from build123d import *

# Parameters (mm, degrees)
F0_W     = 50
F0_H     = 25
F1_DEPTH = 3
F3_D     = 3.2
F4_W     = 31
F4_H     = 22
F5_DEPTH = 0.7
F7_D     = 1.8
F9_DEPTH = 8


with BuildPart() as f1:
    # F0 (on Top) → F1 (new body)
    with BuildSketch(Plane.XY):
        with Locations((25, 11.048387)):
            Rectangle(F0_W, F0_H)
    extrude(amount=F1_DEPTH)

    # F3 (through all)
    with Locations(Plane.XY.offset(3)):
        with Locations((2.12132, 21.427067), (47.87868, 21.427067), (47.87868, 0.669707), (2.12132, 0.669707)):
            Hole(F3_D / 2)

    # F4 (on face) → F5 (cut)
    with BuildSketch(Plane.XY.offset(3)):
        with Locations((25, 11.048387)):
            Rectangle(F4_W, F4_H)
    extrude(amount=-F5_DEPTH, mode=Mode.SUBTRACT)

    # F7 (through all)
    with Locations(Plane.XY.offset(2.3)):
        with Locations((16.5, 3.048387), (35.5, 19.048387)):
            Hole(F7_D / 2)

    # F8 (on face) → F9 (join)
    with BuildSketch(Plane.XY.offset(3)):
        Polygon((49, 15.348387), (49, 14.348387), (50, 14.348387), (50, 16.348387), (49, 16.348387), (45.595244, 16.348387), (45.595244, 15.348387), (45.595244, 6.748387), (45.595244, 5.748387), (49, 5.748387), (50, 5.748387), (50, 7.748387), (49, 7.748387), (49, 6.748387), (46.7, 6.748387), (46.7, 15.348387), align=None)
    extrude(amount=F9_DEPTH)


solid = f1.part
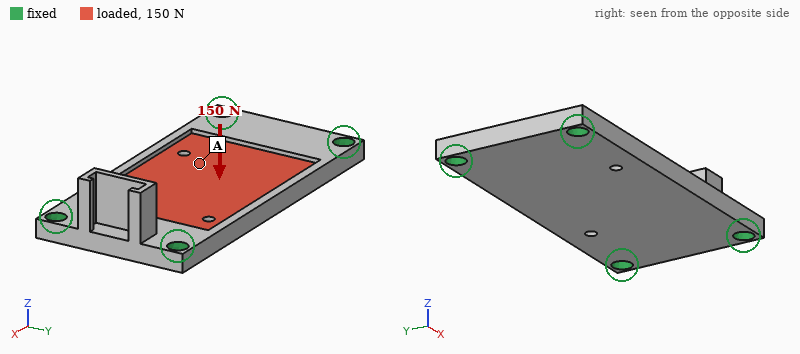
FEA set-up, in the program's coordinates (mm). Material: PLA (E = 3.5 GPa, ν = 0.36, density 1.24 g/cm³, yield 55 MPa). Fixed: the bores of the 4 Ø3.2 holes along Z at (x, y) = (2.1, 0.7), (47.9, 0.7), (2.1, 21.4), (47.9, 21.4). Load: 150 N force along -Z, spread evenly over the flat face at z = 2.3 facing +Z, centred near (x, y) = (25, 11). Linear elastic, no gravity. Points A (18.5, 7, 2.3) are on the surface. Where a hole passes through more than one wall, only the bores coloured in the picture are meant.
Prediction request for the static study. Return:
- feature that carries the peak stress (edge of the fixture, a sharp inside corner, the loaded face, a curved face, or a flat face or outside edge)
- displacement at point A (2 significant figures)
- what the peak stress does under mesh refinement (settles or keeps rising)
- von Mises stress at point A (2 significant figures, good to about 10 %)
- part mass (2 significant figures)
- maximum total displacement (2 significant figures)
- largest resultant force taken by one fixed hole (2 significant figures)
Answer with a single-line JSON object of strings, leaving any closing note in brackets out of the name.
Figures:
{"feature that carries the peak stress": "edge of the fixture", "displacement at point A": "0.33 mm", "what the peak stress does under mesh refinement": "keeps rising", "von Mises stress at point A": "8.0 MPa", "part mass": "4.1 g", "maximum total displacement": "0.39 mm", "largest resultant force taken by one fixed hole": "46 N"}
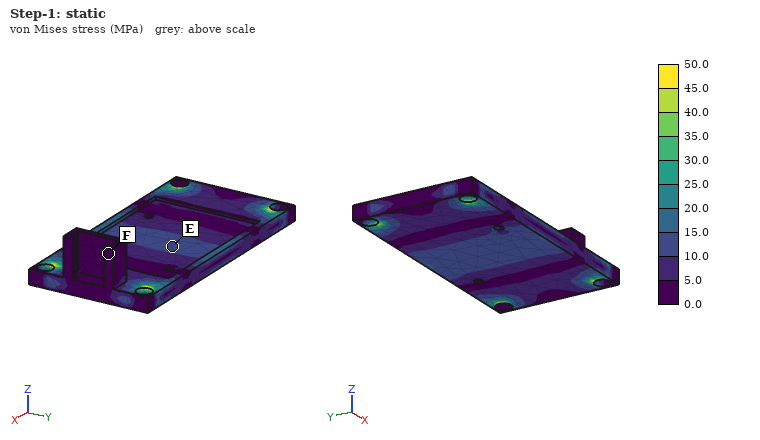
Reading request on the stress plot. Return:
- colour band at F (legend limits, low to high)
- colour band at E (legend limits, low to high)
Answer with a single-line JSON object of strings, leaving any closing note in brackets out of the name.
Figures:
{"colour band at F": "0.0 to 5.0 MPa", "colour band at E": "10.0 to 15.0 MPa"}
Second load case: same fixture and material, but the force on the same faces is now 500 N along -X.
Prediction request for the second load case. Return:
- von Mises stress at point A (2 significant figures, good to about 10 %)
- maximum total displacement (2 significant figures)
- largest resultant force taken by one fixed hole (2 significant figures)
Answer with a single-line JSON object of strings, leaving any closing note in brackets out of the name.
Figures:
{"von Mises stress at point A": "3.2 MPa", "maximum total displacement": "31 µm", "largest resultant force taken by one fixed hole": "130 N"}
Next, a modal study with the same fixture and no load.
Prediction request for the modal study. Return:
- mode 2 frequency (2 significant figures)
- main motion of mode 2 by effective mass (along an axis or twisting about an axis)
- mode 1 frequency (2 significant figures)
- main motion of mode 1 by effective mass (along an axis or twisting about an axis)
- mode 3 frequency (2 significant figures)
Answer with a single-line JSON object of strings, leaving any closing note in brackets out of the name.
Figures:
{"mode 2 frequency": "3500 Hz", "main motion of mode 2 by effective mass": "twisting about X", "mode 1 frequency": "2300 Hz", "main motion of mode 1 by effective mass": "along Z", "mode 3 frequency": "5600 Hz"}
